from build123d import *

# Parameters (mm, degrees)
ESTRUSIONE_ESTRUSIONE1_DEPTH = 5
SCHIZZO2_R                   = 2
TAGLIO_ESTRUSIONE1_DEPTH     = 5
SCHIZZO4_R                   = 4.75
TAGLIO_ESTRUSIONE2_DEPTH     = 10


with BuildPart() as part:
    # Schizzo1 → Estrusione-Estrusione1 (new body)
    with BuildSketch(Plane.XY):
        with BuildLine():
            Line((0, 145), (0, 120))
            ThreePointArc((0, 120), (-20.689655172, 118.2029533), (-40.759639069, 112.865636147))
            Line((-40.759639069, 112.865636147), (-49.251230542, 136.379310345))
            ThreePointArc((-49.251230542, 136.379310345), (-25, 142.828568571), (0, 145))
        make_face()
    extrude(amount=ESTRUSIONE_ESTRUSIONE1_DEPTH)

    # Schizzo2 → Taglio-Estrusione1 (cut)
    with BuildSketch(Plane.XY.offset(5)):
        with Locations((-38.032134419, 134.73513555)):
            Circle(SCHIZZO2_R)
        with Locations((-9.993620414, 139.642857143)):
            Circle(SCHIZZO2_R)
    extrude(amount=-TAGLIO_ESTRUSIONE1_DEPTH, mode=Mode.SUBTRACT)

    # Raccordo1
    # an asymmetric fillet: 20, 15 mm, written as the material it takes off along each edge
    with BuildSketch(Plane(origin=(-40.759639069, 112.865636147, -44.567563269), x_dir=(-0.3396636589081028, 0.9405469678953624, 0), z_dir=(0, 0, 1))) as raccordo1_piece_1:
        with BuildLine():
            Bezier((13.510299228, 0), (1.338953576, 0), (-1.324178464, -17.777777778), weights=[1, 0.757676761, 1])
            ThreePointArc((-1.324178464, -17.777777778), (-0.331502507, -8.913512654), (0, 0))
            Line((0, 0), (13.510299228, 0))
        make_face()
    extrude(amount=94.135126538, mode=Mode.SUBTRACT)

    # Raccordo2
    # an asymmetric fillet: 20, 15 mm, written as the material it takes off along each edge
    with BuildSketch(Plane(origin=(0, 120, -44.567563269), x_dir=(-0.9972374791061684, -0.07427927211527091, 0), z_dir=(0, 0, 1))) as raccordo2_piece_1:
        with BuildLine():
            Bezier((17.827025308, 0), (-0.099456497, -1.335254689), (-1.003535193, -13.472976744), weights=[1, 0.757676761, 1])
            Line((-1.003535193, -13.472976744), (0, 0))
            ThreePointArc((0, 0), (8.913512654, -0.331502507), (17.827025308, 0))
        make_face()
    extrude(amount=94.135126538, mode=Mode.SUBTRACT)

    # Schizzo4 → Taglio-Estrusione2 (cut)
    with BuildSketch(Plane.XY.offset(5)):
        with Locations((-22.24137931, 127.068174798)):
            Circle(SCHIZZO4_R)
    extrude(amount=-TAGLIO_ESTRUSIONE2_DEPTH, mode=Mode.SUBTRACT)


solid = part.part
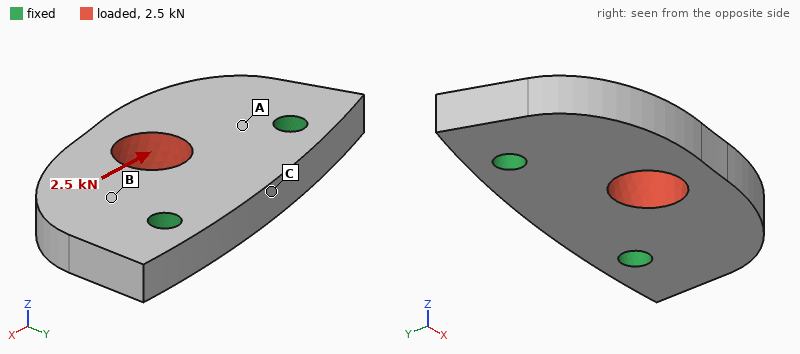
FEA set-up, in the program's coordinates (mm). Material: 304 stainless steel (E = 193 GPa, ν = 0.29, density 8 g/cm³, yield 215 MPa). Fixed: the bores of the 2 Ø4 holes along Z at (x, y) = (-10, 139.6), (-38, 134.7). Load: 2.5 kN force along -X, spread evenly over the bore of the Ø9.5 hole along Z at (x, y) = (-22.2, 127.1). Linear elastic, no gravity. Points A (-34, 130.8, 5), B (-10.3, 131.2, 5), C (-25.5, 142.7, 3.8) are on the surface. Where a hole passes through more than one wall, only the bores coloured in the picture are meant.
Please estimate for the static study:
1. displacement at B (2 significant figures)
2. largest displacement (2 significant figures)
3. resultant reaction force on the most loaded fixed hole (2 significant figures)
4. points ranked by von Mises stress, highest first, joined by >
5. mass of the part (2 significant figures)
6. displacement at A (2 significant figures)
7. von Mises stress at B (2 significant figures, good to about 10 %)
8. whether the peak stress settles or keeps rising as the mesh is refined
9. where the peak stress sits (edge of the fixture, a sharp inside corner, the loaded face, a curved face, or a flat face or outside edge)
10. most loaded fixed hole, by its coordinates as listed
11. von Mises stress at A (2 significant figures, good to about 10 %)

2.0 µm
4.6 µm
1.6 kN
A > B > C
38 g
1.0 µm
15 MPa
keeps rising
edge of the fixture
(-38, 134.7)
30 MPa
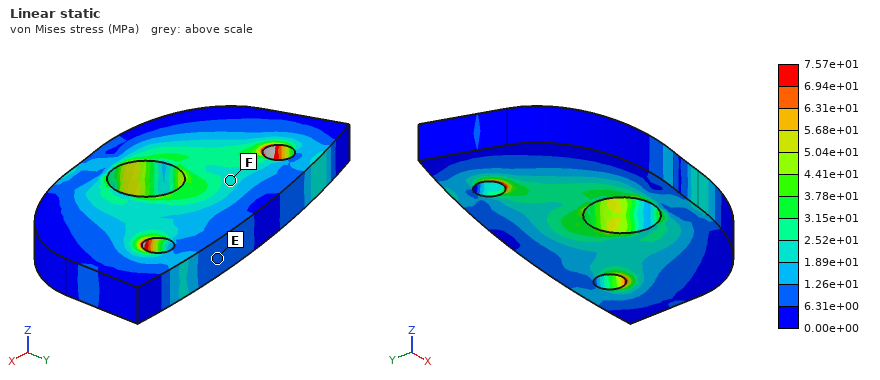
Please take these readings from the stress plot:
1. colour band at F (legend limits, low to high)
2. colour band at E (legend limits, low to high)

1.89e+01 to 2.52e+01 MPa
6.31e+00 to 1.26e+01 MPa
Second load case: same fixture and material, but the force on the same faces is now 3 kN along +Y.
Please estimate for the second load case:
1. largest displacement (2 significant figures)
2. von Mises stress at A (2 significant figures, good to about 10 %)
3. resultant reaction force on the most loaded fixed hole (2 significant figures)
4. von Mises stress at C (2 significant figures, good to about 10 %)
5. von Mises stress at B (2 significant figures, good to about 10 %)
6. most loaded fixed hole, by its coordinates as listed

4.5 µm
30 MPa
1.8 kN
27 MPa
26 MPa
(-10, 139.6)
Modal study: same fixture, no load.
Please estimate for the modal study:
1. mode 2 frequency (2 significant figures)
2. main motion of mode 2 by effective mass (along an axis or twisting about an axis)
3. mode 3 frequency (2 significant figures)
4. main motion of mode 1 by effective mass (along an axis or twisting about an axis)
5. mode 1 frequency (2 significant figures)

18 kHz
twisting about Y
25 kHz
along Z
11 kHz
